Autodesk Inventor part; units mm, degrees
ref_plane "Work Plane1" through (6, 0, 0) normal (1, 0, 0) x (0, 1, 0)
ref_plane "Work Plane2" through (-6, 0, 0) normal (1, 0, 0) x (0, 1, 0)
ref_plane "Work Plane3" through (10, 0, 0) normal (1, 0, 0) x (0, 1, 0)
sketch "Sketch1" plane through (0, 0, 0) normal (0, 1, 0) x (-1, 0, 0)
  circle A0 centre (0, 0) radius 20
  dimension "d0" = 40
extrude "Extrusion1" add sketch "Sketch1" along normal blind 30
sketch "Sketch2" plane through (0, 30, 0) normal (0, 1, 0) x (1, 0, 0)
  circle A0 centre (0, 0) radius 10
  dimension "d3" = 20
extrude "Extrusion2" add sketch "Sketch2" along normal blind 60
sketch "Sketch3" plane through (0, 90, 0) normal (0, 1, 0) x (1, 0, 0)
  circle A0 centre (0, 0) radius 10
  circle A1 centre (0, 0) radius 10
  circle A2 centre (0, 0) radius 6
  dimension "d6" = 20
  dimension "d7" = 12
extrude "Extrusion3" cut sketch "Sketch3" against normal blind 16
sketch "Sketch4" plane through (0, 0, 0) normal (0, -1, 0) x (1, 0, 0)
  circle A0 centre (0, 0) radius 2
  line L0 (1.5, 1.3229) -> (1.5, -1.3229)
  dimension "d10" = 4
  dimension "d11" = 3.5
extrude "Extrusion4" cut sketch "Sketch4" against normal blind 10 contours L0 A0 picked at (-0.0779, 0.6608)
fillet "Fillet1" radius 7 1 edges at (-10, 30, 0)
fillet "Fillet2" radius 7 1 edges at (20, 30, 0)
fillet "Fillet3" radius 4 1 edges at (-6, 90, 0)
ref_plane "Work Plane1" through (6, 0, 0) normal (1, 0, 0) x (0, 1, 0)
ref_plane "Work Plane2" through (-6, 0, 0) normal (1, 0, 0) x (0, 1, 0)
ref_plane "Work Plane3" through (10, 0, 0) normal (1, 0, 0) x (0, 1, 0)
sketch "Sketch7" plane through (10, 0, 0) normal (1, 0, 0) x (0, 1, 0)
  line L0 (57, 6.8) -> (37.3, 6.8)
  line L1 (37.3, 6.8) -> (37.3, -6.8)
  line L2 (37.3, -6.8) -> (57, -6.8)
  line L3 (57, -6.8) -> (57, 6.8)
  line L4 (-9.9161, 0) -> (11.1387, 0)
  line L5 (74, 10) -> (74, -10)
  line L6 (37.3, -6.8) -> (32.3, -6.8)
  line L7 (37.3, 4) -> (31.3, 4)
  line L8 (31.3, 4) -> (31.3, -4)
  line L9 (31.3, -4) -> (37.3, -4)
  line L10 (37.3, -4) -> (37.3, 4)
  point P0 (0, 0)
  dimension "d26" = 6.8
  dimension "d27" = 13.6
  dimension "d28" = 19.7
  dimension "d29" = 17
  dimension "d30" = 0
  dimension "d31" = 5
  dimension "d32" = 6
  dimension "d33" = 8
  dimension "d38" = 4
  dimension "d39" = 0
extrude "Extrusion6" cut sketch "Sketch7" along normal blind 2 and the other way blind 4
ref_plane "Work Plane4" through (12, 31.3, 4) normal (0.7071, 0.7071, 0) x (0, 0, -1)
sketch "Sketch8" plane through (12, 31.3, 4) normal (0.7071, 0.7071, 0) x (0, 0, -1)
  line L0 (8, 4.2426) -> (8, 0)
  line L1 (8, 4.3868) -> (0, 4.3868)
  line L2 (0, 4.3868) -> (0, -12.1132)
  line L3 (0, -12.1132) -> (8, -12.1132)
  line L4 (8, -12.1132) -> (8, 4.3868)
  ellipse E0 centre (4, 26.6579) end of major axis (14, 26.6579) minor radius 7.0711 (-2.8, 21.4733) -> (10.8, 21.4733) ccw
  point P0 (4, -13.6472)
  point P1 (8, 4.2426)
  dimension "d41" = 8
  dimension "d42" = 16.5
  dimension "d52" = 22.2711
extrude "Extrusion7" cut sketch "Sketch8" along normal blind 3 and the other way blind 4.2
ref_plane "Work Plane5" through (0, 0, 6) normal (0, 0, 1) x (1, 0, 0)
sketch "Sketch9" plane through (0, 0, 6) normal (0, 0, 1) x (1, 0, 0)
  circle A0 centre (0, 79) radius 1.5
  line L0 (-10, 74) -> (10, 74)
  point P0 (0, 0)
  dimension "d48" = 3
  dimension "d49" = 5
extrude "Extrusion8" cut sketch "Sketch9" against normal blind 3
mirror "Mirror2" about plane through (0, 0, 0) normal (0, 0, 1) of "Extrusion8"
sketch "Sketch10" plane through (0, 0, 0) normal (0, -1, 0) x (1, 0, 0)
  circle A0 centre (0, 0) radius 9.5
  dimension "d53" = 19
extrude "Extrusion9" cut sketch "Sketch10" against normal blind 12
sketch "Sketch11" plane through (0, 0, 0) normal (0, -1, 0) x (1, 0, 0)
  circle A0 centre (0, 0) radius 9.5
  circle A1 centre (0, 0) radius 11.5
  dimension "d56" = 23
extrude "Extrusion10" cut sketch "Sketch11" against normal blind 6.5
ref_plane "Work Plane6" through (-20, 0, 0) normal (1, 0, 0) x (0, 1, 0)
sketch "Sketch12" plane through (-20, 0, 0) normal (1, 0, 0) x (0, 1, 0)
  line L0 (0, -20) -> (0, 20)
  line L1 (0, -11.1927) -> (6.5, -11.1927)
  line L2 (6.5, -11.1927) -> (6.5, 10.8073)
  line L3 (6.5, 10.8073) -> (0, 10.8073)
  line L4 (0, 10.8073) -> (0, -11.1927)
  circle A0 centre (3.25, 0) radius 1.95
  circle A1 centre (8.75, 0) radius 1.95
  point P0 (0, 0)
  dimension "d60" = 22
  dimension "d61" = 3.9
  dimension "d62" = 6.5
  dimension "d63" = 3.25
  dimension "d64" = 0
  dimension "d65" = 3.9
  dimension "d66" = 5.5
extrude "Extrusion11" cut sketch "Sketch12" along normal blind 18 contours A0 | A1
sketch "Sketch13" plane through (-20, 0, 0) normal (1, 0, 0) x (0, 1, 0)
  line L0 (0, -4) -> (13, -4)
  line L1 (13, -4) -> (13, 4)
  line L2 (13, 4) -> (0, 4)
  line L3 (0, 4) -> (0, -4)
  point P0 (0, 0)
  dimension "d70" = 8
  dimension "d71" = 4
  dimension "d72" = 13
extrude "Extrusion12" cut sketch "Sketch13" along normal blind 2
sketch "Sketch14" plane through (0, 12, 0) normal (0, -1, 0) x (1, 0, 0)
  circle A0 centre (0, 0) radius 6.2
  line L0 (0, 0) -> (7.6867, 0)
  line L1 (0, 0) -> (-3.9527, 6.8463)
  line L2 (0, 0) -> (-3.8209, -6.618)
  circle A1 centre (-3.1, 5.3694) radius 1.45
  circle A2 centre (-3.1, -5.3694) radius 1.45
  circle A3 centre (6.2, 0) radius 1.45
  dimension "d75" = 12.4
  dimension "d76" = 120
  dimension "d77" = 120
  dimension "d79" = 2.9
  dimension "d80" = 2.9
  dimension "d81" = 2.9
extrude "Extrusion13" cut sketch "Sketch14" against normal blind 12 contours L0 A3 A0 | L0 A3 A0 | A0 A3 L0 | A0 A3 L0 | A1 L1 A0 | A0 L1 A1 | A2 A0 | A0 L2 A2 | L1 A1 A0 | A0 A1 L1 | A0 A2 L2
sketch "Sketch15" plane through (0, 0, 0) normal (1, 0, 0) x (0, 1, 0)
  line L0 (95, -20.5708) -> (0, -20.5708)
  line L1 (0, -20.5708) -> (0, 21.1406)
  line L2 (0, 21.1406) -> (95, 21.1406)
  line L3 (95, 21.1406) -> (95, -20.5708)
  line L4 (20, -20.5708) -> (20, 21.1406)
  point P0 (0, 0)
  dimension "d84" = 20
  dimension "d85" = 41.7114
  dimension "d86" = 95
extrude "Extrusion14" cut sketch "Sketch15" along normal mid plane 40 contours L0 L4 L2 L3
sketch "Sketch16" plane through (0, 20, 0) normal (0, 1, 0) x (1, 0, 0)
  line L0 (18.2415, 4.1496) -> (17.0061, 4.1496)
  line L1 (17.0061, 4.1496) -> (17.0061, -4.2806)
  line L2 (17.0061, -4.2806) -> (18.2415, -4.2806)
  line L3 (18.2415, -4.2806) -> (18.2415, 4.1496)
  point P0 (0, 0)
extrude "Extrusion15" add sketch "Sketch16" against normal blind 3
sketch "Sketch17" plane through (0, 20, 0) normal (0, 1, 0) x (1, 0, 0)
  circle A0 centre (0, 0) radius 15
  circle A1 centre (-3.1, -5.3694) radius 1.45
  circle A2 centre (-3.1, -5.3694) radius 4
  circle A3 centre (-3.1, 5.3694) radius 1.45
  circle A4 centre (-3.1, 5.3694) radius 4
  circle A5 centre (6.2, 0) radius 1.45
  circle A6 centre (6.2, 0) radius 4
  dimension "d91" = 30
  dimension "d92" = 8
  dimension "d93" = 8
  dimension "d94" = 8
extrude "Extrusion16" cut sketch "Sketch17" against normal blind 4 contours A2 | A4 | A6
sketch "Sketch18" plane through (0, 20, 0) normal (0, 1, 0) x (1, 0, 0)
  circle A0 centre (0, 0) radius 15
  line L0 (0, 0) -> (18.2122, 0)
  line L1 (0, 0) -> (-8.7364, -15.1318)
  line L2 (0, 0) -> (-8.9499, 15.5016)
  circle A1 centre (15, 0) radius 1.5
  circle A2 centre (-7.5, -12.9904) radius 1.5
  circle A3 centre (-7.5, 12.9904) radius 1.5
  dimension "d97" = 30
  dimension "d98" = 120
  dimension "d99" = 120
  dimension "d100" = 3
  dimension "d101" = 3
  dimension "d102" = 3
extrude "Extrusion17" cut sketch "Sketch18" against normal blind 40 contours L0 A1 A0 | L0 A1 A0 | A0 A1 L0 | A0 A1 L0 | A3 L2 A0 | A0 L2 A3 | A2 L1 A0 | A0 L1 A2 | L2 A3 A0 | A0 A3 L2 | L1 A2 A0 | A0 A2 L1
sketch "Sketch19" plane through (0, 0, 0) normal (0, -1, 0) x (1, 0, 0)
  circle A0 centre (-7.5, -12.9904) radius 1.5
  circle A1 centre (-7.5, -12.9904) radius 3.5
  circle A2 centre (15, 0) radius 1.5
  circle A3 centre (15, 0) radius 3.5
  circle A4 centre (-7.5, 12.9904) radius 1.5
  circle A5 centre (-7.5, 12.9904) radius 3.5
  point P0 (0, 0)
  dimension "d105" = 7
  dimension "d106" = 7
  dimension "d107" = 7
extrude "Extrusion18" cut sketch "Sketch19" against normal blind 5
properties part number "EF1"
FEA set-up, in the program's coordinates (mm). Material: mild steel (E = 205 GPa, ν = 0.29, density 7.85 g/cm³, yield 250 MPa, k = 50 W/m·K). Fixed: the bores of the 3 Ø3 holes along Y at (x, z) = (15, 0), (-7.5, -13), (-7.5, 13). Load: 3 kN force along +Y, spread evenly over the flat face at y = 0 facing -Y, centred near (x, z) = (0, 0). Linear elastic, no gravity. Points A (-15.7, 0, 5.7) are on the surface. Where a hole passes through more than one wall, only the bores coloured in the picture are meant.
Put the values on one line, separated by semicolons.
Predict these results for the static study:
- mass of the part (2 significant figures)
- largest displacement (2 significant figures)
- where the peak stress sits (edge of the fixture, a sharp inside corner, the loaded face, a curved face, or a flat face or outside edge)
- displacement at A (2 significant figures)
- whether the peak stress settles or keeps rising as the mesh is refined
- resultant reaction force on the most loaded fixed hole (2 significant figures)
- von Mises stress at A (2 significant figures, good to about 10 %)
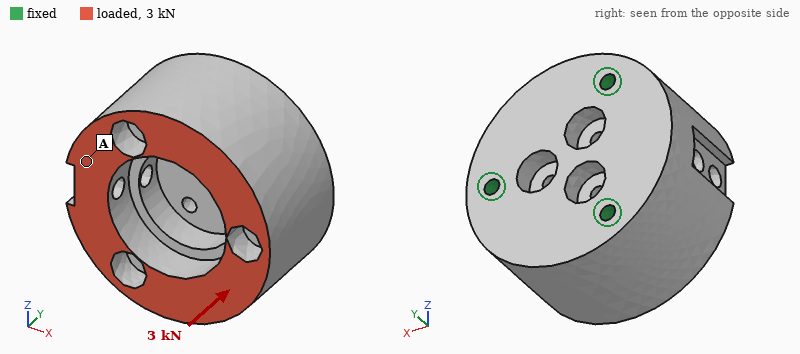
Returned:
150 g; 1.1 µm; a sharp inside corner; 0.76 µm; keeps rising; 1.0 kN; 4.3 MPa
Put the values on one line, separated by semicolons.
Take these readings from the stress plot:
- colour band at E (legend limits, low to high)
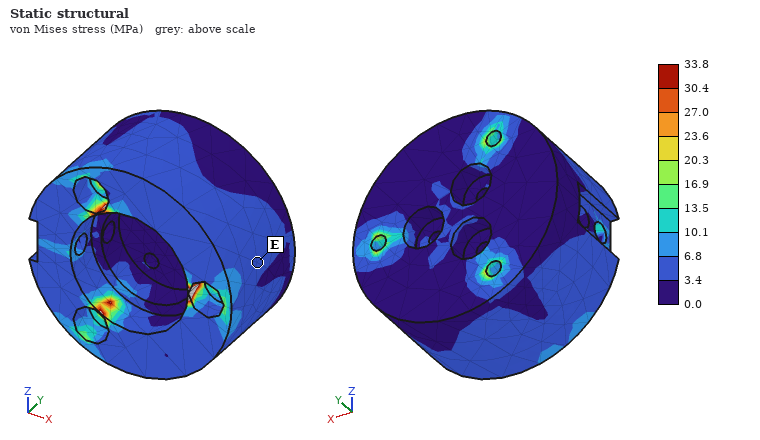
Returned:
3.4 to 6.8 MPa
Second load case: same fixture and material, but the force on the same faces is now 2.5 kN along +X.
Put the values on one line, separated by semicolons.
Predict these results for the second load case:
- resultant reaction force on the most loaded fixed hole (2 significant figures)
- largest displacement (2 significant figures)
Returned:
1.1 kN; 2.7 µm
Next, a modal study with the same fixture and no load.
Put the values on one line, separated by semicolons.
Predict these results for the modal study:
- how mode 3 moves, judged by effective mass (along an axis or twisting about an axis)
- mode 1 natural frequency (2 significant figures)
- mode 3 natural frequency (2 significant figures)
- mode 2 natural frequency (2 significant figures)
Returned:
along Y; 29 kHz; 35 kHz; 30 kHz
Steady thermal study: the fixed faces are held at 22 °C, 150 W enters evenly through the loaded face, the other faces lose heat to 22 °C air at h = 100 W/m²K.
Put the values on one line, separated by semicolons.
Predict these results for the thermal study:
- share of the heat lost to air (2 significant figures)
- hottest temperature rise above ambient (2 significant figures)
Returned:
8.6 %; 66 K
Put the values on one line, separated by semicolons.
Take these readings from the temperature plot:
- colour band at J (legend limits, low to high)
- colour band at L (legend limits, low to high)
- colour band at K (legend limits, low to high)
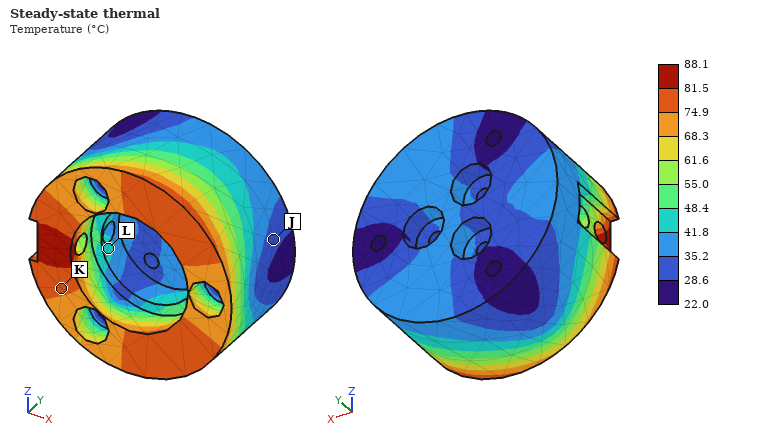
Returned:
28.6 to 35.2 °C; 41.8 to 48.4 °C; 74.9 to 81.5 °C
